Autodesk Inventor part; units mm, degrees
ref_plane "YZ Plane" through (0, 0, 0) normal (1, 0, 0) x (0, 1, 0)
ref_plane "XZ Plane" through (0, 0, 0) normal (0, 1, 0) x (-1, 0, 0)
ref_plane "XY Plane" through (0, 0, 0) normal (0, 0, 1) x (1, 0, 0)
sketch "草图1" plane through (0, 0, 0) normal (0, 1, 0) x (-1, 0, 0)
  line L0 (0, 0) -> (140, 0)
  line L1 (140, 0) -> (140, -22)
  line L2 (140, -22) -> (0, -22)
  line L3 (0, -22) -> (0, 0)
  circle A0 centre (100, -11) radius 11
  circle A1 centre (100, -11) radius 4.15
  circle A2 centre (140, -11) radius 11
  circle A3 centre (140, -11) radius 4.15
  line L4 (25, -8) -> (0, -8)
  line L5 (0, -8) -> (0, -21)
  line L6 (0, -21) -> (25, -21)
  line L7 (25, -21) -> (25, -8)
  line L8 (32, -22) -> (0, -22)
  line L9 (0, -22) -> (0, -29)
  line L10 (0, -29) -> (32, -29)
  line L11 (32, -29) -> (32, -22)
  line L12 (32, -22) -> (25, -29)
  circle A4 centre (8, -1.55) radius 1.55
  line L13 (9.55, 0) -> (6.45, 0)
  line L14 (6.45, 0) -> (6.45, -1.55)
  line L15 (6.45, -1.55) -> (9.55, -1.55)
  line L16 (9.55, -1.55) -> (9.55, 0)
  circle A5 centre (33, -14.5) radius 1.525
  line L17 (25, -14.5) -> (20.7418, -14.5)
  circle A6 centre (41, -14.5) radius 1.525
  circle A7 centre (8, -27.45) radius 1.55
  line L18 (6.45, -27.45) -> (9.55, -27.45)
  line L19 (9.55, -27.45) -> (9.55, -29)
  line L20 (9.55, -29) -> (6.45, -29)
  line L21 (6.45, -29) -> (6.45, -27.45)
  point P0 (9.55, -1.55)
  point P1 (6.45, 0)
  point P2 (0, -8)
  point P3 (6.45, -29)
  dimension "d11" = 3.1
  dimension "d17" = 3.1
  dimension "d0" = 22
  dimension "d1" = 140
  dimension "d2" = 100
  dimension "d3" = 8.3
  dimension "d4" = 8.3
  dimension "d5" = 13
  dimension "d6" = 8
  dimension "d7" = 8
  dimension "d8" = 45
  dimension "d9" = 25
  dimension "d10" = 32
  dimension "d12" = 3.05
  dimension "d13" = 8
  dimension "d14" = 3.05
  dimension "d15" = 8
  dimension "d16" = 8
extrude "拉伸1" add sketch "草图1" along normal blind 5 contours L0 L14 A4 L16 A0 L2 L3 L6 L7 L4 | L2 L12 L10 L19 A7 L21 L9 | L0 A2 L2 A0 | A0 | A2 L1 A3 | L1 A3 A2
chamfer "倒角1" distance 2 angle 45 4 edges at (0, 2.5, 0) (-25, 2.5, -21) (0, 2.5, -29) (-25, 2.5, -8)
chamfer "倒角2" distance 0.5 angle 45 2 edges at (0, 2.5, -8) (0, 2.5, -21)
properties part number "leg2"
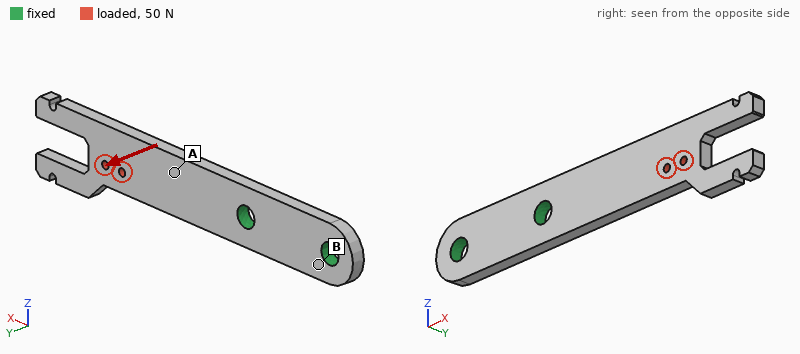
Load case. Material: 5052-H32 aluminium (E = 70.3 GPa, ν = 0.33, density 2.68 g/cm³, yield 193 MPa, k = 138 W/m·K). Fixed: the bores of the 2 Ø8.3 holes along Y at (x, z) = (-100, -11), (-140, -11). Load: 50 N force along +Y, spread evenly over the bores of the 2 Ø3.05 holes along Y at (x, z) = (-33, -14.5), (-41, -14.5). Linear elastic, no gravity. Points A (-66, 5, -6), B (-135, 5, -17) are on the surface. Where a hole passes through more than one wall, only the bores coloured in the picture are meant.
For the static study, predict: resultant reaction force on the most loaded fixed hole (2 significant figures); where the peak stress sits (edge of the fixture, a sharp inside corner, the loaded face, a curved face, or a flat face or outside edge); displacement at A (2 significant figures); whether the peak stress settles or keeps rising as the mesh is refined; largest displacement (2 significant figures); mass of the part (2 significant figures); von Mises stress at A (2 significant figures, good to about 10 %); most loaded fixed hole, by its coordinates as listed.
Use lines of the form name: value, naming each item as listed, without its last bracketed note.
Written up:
resultant reaction force on the most loaded fixed hole: 50 N
where the peak stress sits: edge of the fixture
displacement at A: 0.075 mm
whether the peak stress settles or keeps rising as the mesh is refined: keeps rising
largest displacement: 0.44 mm
mass of the part: 40 g
von Mises stress at A: 16 MPa
most loaded fixed hole, by its coordinates as listed: (-100, -11)
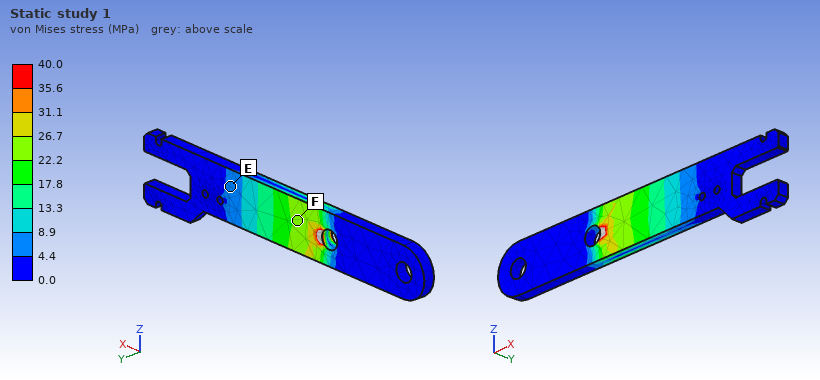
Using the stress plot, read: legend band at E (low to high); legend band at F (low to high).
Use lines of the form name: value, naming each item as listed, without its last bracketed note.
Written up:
legend band at E: 4.4 to 8.9 MPa
legend band at F: 22.2 to 26.7 MPa
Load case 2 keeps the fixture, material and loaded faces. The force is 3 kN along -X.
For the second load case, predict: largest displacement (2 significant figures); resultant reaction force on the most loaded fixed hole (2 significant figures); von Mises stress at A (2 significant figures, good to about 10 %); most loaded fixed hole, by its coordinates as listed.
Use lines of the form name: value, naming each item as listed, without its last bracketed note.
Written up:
largest displacement: 0.17 mm
resultant reaction force on the most loaded fixed hole: 2.9 kN
von Mises stress at A: 15 MPa
most loaded fixed hole, by its coordinates as listed: (-100, -11)
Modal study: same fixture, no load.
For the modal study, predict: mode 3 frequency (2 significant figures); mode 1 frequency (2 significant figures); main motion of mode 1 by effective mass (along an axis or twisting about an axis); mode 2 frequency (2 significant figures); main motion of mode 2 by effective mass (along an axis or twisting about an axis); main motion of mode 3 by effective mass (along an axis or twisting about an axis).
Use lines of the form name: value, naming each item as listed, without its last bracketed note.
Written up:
mode 3 frequency: 2300 Hz
mode 1 frequency: 490 Hz
main motion of mode 1 by effective mass: along Y
mode 2 frequency: 1800 Hz
main motion of mode 2 by effective mass: along Z
main motion of mode 3 by effective mass: twisting about X
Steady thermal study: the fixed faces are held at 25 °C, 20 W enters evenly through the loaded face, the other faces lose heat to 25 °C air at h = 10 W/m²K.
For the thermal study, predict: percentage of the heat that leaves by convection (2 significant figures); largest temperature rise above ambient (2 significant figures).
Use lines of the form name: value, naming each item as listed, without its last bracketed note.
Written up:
percentage of the heat that leaves by convection: 13 %
largest temperature rise above ambient: 76 K
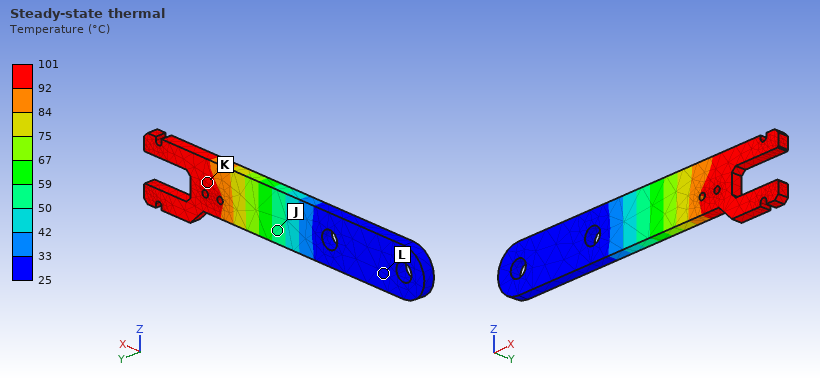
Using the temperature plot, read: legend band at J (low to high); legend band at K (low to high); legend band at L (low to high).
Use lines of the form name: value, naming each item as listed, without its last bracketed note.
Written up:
legend band at J: 50 to 59 °C
legend band at K: 92 to 101 °C
legend band at L: 25 to 33 °C
